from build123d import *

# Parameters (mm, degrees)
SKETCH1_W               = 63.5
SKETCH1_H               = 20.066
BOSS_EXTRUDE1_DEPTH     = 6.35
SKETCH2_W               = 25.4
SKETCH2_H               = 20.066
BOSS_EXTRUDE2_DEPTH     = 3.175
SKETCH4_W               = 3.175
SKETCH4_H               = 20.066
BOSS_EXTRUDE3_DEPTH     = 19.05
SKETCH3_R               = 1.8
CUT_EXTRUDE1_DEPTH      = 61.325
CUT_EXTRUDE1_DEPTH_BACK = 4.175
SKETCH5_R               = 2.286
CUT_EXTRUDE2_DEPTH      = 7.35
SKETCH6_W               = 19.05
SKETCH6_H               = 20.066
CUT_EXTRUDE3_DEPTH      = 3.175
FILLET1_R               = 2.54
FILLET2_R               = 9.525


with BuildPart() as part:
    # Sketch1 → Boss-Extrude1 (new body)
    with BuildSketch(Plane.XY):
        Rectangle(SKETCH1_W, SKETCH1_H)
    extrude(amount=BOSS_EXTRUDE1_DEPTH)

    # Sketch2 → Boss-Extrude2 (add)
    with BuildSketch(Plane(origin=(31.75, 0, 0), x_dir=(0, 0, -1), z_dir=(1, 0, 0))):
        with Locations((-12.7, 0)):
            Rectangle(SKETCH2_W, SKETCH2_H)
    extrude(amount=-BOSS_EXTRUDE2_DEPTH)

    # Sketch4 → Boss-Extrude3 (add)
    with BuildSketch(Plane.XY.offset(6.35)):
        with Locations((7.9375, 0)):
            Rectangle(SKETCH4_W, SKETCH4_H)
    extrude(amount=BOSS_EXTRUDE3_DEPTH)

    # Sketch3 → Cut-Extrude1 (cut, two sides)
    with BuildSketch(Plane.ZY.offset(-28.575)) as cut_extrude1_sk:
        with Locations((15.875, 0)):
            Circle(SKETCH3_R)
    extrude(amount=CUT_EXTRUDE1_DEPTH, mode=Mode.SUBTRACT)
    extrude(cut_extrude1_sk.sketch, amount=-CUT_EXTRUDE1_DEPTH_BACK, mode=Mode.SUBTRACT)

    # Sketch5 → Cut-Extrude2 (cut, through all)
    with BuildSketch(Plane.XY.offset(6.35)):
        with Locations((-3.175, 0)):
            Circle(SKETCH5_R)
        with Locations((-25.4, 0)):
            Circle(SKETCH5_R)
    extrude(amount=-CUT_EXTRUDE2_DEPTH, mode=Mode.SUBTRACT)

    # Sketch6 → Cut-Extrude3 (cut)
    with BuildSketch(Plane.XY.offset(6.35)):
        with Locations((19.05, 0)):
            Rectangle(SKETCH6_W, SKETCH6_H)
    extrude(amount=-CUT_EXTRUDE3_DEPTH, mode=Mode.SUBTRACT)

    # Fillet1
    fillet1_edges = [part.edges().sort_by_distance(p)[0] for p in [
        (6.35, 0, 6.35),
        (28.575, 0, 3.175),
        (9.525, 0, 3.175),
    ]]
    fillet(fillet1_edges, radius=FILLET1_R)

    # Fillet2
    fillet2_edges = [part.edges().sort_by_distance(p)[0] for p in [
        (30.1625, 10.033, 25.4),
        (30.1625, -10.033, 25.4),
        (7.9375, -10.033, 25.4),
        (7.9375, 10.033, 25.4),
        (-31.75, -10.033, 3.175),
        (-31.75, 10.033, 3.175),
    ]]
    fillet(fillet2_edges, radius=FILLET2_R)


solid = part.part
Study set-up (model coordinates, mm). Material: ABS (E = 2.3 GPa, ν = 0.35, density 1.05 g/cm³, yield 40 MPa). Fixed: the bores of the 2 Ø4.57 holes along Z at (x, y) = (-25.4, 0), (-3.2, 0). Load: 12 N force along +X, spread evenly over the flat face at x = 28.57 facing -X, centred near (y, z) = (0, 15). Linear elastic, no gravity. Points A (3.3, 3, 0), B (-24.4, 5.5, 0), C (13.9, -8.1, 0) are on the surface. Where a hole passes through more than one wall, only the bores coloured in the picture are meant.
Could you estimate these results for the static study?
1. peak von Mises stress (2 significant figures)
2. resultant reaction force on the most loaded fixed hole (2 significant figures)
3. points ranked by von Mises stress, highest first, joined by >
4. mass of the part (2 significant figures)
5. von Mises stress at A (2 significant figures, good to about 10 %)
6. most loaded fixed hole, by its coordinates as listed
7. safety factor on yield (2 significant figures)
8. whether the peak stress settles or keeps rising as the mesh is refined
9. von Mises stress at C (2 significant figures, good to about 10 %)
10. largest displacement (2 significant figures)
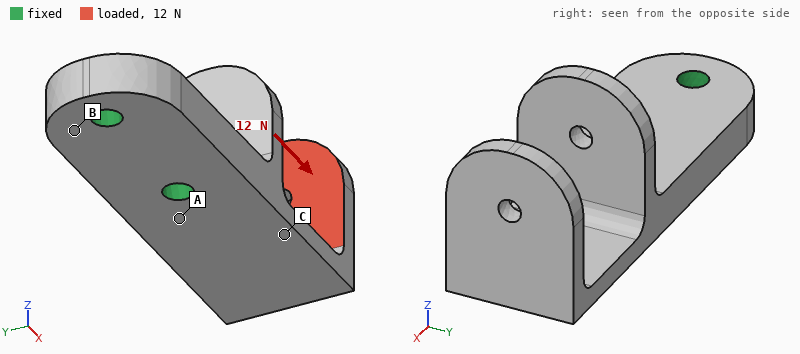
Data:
5.4 MPa
11 N
C > A > B
9.1 g
0.92 MPa
(-3.2, 0)
7.5
settles
4.3 MPa
0.79 mm
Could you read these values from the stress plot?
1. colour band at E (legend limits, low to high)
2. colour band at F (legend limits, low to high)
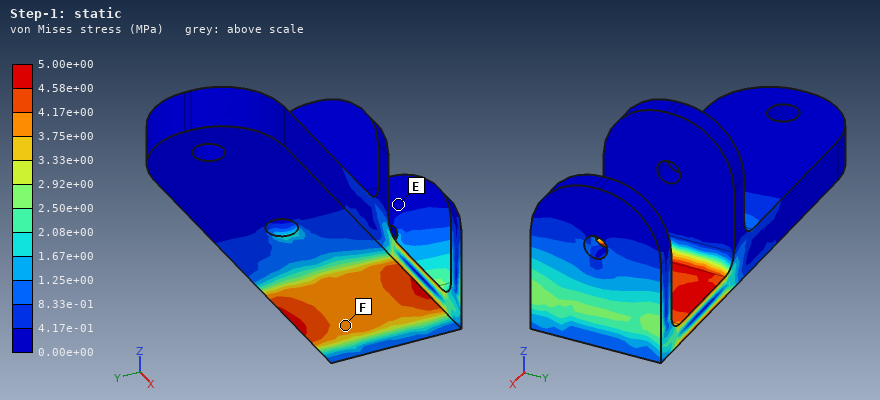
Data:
0.00e+00 to 4.17e-01 MPa
3.75e+00 to 4.17e+00 MPa
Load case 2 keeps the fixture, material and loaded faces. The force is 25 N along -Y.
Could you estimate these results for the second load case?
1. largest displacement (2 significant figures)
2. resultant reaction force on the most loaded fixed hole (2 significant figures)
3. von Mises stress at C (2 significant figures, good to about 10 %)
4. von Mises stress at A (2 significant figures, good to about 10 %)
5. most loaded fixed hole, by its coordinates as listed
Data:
0.82 mm
48 N
6.8 MPa
2.4 MPa
(-3.2, 0)
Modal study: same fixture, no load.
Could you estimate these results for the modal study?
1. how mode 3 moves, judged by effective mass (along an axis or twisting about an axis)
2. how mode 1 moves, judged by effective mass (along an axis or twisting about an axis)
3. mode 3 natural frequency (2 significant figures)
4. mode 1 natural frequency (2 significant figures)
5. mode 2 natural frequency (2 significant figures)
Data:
along Z
along Z
1400 Hz
530 Hz
900 Hz
